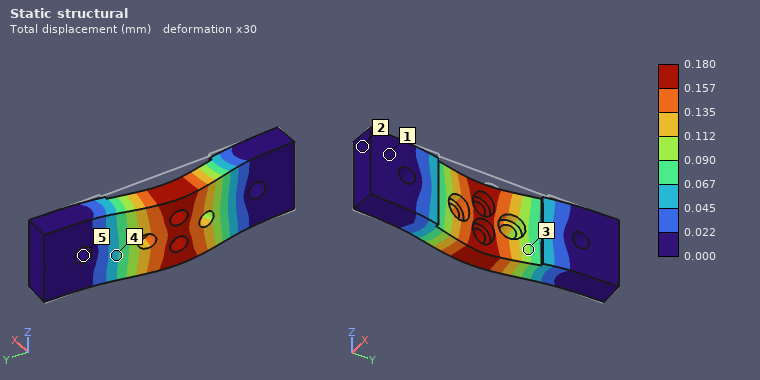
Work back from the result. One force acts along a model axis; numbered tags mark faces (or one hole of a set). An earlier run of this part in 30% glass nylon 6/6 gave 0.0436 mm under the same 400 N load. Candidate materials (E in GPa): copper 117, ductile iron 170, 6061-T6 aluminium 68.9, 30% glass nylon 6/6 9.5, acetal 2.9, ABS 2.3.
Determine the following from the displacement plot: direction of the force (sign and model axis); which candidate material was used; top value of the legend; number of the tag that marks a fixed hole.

-X
ABS
0.180 mm
5
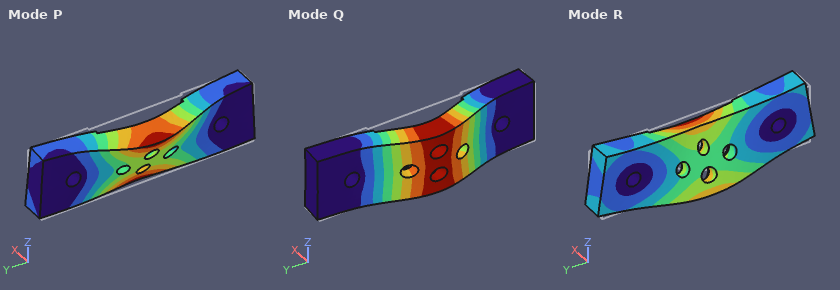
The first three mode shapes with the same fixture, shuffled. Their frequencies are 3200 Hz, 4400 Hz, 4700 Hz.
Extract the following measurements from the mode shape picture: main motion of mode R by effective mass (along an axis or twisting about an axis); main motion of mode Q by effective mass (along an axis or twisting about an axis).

along Z
along X
